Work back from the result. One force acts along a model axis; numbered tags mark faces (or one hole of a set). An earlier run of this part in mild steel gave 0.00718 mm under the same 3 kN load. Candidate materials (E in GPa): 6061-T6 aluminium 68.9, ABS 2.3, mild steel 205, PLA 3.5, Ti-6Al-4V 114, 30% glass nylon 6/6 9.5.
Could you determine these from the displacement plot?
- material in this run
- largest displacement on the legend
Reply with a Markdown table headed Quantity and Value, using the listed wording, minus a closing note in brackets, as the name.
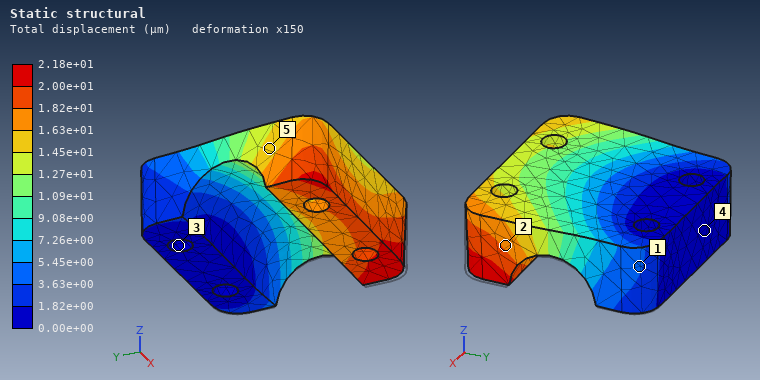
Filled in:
| Quantity | Value |
|---|---|
| material in this run | 6061-T6 aluminium |
| largest displacement on the legend | 2.18e+01 µm |
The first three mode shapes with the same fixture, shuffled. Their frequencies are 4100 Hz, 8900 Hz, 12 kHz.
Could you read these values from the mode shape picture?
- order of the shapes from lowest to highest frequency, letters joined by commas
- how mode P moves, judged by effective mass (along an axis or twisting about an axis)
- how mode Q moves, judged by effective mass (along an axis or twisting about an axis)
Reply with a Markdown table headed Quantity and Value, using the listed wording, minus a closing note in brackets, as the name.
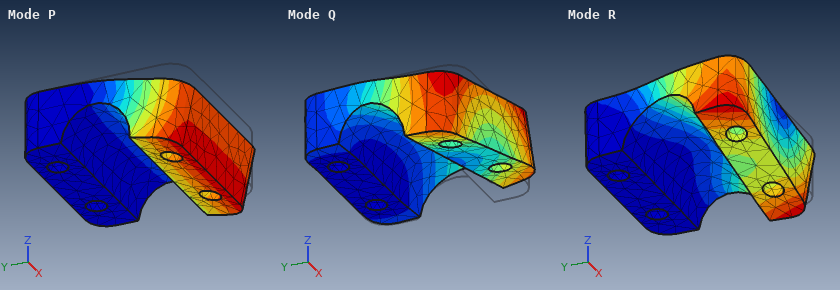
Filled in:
| Quantity | Value |
|---|---|
| order of the shapes from lowest to highest frequency, letters joined by commas | P, R, Q |
| how mode P moves, judged by effective mass | along Z |
| how mode Q moves, judged by effective mass | along X |
